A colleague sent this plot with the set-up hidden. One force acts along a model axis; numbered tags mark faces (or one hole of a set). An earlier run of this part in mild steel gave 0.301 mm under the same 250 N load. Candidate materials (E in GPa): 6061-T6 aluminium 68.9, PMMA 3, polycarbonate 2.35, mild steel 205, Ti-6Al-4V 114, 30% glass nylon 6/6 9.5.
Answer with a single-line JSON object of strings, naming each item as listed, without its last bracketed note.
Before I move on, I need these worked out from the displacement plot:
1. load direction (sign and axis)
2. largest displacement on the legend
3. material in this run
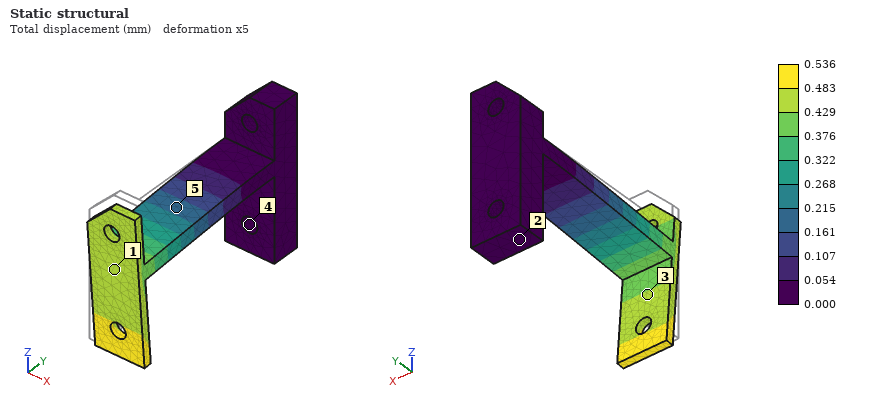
{"load direction": "-Z", "largest displacement on the legend": "0.536 mm", "material in this run": "Ti-6Al-4V"}
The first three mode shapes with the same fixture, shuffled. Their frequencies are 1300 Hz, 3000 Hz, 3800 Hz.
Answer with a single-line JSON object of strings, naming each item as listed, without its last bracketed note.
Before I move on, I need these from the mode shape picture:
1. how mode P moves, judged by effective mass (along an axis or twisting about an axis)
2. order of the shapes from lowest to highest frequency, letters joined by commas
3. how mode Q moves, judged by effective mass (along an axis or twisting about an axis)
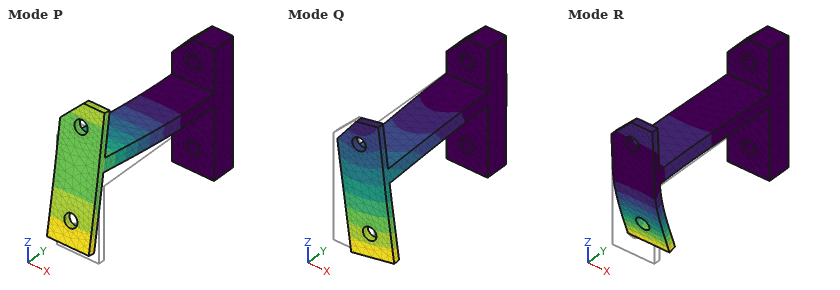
{"how mode P moves, judged by effective mass": "along Z", "order of the shapes from lowest to highest frequency, letters joined by commas": "P, Q, R", "how mode Q moves, judged by effective mass": "along X"}
